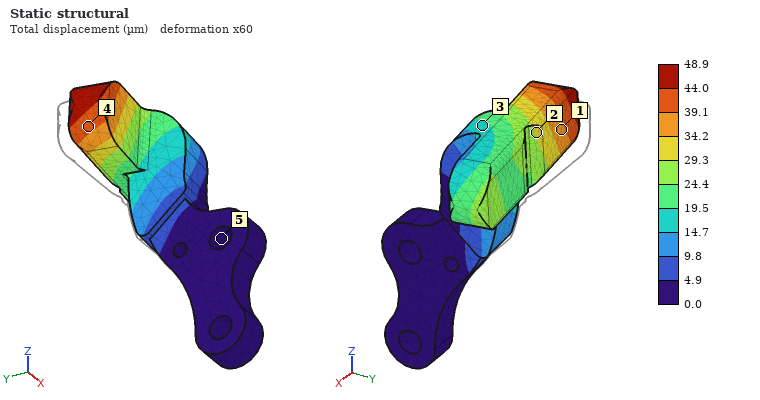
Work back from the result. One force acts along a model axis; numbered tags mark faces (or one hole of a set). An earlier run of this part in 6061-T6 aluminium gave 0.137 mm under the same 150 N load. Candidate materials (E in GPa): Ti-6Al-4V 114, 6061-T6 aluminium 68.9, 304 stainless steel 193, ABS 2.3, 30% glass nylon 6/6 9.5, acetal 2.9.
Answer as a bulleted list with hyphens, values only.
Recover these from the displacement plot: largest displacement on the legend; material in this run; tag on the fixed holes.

- 48.9 µm
- 304 stainless steel
- 5
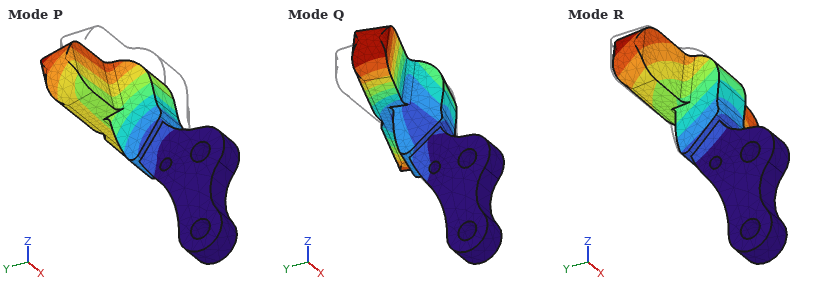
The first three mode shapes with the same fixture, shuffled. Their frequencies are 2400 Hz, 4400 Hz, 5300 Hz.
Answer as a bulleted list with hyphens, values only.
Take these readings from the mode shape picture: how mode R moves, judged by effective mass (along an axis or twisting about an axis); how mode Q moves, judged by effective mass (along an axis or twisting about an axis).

- along X
- twisting about Z
